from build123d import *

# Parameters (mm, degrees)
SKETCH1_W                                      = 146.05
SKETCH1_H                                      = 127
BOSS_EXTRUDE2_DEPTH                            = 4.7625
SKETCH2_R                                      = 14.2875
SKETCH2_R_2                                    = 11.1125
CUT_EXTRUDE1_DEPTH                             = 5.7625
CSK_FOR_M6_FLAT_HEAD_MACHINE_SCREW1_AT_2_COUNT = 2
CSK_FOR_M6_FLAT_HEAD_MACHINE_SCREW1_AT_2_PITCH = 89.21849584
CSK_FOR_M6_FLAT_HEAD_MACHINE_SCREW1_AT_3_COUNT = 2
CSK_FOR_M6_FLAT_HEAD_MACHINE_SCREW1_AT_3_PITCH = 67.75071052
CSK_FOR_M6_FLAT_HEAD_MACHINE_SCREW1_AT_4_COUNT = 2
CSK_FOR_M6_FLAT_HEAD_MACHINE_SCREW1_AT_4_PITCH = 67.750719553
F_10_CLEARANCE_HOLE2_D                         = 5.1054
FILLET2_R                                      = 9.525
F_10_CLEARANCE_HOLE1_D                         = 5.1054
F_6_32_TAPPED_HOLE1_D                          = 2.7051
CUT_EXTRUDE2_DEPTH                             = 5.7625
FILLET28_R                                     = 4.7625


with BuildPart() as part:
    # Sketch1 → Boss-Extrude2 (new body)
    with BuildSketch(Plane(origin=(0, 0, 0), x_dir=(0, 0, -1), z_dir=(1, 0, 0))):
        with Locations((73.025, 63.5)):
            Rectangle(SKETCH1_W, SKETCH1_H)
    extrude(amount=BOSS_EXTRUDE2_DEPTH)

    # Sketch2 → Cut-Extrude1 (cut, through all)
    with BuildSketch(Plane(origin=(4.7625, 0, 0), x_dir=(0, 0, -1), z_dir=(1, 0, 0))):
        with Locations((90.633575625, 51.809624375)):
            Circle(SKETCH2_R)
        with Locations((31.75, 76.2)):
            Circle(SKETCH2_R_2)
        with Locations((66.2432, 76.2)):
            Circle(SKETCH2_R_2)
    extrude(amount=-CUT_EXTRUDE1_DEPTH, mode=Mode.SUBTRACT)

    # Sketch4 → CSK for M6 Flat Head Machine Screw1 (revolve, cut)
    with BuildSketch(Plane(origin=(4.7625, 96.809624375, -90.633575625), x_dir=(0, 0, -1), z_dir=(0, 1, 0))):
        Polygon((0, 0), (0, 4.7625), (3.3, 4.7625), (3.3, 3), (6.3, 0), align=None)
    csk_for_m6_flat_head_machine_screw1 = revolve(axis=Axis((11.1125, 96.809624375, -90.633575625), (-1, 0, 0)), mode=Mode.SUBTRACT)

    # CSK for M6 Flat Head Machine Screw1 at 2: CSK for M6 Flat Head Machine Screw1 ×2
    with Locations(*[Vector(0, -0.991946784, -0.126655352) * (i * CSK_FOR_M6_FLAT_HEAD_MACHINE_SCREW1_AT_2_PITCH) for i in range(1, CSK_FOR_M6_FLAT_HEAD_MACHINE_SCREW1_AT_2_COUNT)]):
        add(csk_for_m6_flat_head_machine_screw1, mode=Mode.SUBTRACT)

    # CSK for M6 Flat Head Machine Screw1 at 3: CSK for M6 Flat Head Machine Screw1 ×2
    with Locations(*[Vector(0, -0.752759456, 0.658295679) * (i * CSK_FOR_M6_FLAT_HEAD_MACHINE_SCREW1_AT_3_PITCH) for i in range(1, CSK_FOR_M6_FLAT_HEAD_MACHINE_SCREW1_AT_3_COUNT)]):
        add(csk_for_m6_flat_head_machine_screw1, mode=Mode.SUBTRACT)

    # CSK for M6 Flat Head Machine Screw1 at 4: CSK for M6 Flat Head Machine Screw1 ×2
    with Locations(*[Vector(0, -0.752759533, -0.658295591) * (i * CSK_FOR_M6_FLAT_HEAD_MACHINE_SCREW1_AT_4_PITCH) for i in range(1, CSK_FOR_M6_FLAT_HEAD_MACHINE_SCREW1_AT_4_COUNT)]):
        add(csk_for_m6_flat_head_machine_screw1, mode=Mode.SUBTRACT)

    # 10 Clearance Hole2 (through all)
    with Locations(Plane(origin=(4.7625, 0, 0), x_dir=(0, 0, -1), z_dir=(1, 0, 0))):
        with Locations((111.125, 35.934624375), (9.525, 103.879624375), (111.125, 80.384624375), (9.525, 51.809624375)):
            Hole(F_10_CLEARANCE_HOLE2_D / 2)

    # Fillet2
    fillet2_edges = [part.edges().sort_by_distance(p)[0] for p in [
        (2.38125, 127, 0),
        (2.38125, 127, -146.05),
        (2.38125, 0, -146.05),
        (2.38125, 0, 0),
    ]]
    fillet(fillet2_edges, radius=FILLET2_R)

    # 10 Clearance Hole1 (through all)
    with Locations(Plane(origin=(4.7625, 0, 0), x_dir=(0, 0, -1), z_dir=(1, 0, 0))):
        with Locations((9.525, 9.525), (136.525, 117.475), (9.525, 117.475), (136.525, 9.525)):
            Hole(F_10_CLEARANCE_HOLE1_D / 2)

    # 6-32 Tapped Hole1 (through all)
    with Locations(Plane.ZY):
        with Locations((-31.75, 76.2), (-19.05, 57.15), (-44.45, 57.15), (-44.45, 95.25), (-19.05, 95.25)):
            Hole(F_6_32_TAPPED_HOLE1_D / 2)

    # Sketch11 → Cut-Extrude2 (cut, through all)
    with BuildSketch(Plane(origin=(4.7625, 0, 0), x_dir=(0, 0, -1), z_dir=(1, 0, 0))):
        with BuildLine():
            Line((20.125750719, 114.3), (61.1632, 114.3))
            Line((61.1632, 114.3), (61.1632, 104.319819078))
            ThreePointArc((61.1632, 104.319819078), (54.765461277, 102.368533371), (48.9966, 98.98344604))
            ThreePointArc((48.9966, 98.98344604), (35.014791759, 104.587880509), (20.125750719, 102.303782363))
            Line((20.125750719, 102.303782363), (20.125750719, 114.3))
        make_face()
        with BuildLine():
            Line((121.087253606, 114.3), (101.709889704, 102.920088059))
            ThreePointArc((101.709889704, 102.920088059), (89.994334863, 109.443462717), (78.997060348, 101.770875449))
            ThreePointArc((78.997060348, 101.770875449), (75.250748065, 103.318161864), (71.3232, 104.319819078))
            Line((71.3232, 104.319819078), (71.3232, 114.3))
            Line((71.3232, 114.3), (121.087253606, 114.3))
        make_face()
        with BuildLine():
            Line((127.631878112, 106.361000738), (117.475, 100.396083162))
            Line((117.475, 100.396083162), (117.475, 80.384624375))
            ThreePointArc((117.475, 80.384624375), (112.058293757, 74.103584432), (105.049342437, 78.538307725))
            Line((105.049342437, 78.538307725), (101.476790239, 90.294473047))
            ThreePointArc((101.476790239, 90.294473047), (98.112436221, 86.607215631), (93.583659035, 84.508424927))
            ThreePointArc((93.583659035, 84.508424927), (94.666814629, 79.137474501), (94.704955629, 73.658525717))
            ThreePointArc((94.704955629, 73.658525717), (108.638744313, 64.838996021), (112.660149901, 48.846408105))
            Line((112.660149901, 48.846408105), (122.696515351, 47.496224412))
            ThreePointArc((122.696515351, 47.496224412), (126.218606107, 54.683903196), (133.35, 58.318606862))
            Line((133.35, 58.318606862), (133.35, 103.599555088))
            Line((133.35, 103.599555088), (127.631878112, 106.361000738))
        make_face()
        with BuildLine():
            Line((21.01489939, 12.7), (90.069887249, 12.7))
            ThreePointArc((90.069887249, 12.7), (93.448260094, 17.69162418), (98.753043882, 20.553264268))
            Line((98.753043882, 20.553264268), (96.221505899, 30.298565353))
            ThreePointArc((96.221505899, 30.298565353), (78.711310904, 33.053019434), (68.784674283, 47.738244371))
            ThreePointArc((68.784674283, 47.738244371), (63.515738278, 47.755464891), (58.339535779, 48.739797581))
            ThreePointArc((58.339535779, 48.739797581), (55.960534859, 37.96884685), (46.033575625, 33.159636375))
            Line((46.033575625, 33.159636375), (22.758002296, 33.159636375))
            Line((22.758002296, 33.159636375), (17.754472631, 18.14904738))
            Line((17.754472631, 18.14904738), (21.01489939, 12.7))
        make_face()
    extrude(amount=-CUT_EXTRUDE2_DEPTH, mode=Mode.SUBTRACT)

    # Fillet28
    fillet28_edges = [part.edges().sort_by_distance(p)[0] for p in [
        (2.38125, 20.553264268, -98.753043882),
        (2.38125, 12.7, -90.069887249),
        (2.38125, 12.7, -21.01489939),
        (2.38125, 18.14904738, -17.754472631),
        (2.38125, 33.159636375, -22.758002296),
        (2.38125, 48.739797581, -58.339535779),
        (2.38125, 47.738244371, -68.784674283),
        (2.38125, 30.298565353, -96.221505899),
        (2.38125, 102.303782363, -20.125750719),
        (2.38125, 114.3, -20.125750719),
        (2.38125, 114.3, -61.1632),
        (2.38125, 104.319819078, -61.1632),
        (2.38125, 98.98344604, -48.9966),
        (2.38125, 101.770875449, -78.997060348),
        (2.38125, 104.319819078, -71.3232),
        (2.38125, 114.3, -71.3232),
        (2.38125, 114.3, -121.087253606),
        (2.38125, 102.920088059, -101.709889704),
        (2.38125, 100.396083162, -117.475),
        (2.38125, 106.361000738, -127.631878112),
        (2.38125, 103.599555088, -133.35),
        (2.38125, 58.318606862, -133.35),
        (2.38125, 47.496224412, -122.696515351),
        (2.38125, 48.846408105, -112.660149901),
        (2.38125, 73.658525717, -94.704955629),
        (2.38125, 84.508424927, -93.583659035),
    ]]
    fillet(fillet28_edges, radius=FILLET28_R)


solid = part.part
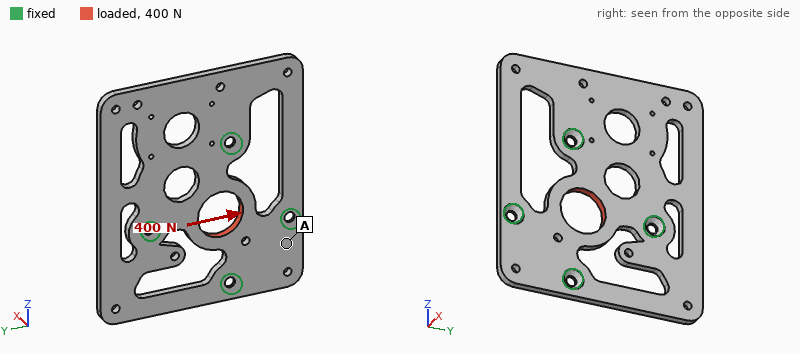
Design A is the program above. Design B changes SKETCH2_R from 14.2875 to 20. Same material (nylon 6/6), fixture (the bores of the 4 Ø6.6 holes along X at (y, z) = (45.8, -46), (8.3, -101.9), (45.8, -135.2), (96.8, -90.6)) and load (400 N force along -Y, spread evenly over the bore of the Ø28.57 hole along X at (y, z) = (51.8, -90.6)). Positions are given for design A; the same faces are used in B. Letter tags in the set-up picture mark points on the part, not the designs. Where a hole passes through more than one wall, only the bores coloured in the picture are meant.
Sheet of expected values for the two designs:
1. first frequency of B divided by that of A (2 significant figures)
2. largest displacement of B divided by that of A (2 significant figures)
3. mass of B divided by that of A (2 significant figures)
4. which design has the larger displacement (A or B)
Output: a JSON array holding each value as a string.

["0.98", "2.7", "0.95", "B"]
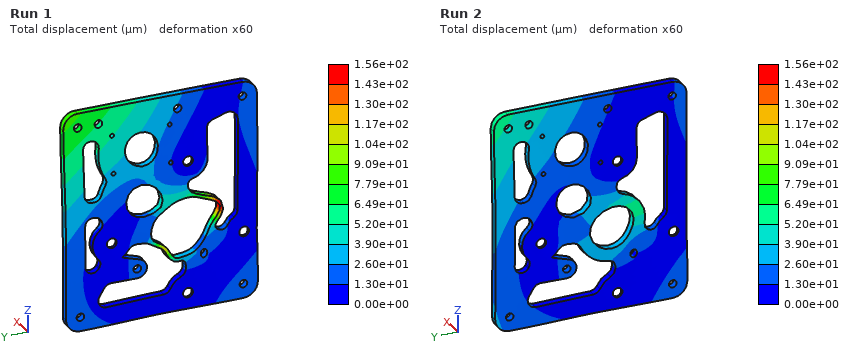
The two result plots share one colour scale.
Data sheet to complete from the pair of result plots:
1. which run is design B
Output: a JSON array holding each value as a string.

["Run 1"]
